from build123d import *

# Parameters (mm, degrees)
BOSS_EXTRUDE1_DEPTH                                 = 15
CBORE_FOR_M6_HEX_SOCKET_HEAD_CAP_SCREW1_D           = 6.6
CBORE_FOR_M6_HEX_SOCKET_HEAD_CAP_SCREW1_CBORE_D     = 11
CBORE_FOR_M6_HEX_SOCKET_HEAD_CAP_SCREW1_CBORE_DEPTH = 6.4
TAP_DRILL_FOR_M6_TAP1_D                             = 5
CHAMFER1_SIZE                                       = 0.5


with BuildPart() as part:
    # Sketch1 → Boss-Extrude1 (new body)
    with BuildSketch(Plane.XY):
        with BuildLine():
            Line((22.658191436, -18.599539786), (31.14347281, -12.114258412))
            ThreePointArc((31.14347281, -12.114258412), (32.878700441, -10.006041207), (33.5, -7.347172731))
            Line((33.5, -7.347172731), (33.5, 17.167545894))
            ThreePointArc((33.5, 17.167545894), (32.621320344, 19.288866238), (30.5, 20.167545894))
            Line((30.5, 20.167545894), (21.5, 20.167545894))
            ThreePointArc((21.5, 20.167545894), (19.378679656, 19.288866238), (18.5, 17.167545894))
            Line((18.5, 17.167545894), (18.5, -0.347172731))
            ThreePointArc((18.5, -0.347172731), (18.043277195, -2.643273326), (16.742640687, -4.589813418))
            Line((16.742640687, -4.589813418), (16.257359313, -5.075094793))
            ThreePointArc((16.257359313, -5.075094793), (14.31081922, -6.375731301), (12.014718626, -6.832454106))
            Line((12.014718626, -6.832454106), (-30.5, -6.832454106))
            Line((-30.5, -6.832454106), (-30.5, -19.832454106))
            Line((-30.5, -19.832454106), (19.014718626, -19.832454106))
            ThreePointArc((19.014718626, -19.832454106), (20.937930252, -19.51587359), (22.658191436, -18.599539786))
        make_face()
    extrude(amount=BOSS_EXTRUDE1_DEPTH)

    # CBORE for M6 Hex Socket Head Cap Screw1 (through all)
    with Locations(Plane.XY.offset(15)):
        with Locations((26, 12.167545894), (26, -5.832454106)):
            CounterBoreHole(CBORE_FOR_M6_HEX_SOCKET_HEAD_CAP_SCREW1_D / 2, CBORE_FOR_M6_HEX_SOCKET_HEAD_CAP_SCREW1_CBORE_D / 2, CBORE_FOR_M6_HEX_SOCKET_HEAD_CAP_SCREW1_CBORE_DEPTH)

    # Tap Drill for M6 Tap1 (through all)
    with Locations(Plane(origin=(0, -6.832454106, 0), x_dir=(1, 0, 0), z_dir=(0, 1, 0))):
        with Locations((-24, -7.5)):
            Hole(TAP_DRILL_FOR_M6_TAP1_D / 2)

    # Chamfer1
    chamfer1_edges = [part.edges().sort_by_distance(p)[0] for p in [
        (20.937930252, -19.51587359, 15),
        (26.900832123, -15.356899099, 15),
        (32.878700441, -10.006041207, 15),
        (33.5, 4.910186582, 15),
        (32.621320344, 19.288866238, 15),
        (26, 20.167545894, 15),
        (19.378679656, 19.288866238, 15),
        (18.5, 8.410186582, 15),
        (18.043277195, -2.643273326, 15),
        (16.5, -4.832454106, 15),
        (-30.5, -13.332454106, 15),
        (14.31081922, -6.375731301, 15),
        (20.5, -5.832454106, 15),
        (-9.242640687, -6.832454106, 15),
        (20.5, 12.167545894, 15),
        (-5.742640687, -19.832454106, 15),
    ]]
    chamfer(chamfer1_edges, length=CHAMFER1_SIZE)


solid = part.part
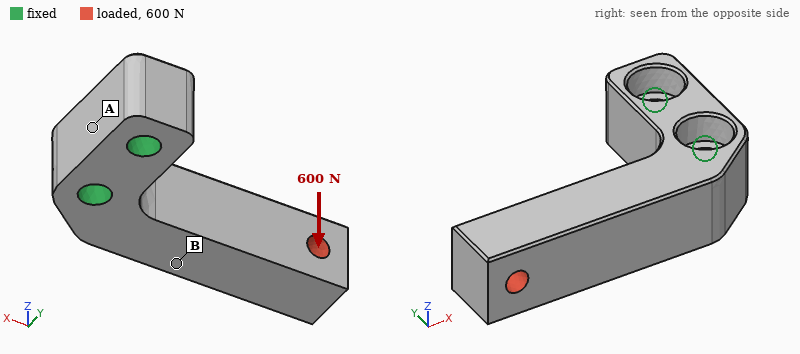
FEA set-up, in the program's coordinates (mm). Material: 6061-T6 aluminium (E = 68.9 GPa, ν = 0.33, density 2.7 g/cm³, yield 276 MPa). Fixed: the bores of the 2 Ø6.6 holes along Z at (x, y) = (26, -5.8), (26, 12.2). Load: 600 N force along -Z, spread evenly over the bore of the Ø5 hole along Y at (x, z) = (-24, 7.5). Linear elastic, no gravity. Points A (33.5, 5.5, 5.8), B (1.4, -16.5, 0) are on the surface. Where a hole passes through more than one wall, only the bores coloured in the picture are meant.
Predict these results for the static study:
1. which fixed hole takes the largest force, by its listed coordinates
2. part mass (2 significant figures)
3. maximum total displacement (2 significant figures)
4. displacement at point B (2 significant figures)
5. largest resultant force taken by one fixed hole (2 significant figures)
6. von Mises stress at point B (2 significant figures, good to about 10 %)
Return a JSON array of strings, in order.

["(26, -5.8)", "42 g", "0.20 mm", "0.065 mm", "790 N", "31 MPa"]
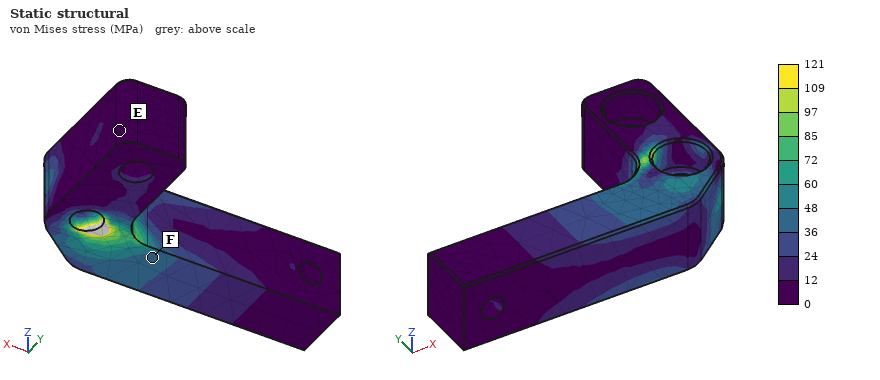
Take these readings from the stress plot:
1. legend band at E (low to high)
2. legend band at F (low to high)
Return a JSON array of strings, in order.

["0 to 12 MPa", "36 to 48 MPa"]
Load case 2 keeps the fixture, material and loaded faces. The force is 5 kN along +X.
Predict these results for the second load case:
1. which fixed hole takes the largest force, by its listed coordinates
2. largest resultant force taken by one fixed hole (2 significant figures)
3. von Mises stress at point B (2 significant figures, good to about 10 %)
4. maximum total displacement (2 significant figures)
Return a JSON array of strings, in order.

["(26, -5.8)", "5.7 kN", "25 MPa", "0.11 mm"]
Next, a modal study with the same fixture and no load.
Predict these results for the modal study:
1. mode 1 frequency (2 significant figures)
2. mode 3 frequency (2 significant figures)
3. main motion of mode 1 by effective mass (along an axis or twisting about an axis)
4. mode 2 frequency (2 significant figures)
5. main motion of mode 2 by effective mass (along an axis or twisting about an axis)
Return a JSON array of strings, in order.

["2900 Hz", "12 kHz", "along Z", "3200 Hz", "along Y"]
